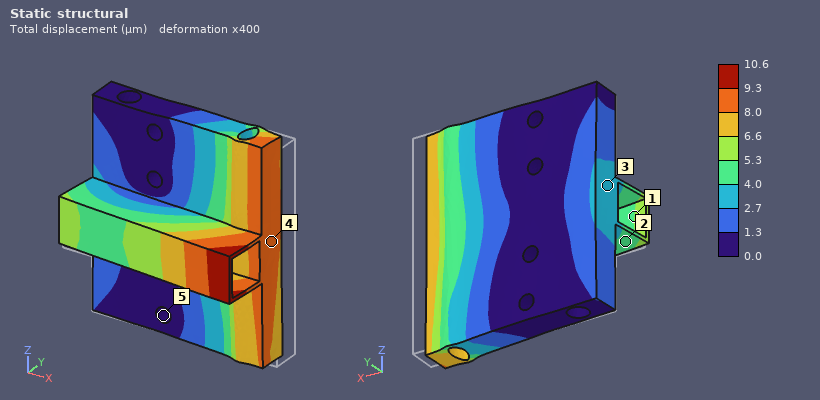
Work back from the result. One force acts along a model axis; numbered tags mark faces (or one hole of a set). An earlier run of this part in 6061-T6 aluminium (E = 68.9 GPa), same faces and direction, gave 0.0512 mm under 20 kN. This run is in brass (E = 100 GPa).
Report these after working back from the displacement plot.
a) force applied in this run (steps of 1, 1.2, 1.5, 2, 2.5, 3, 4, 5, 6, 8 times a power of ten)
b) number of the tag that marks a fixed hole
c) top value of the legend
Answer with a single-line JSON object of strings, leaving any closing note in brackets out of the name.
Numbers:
{"force applied in this run": "6 kN", "number of the tag that marks a fixed hole": "5", "top value of the legend": "10.6 µm"}
